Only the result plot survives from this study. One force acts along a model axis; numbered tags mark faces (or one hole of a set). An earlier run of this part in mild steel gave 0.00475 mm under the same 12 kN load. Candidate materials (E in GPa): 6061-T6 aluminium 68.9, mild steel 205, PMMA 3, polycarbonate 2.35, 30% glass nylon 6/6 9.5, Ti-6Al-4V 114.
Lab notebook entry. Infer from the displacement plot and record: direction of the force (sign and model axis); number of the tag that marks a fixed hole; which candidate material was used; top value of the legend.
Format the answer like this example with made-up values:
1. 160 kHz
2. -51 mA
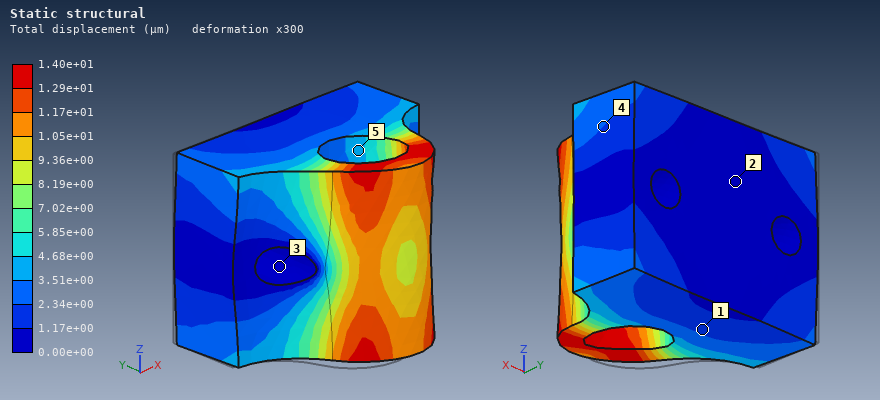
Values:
1. +X
2. 3
3. 6061-T6 aluminium
4. 1.40e+01 µm
